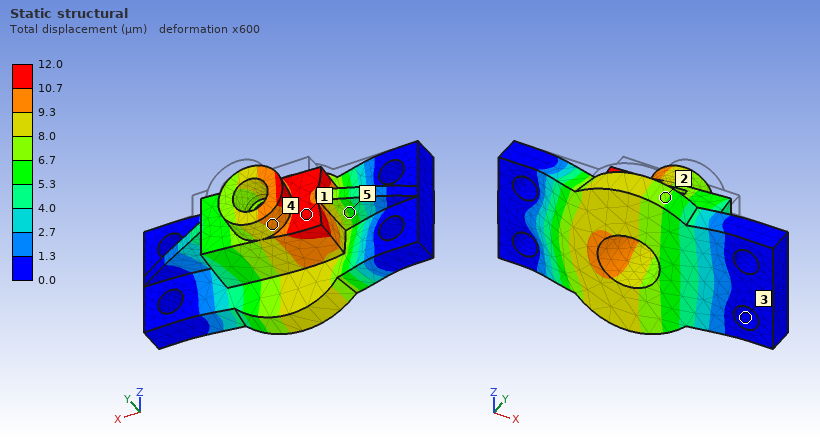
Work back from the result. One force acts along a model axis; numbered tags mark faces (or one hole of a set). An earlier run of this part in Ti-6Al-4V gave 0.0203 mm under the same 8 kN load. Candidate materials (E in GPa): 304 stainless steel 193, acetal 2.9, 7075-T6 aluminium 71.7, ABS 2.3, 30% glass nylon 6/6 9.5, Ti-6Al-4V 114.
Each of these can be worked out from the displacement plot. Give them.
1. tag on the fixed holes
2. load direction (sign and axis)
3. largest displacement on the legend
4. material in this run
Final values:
3
-Y
12.0 µm
304 stainless steel
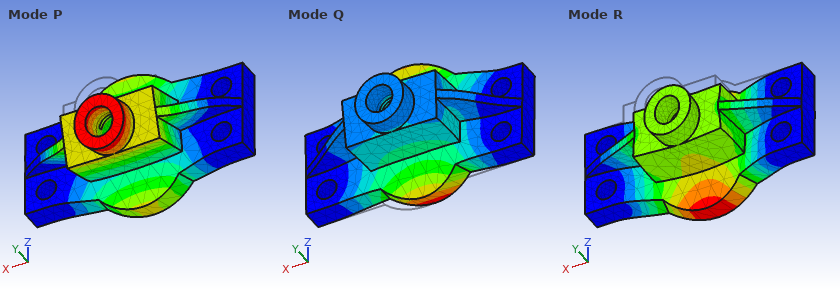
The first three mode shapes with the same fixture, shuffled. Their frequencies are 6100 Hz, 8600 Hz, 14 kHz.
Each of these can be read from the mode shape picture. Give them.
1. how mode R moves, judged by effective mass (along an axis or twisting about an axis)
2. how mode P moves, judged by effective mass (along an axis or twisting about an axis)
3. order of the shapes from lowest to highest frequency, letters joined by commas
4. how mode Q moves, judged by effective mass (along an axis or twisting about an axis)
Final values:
along Y
along Z
P, R, Q
along Z
